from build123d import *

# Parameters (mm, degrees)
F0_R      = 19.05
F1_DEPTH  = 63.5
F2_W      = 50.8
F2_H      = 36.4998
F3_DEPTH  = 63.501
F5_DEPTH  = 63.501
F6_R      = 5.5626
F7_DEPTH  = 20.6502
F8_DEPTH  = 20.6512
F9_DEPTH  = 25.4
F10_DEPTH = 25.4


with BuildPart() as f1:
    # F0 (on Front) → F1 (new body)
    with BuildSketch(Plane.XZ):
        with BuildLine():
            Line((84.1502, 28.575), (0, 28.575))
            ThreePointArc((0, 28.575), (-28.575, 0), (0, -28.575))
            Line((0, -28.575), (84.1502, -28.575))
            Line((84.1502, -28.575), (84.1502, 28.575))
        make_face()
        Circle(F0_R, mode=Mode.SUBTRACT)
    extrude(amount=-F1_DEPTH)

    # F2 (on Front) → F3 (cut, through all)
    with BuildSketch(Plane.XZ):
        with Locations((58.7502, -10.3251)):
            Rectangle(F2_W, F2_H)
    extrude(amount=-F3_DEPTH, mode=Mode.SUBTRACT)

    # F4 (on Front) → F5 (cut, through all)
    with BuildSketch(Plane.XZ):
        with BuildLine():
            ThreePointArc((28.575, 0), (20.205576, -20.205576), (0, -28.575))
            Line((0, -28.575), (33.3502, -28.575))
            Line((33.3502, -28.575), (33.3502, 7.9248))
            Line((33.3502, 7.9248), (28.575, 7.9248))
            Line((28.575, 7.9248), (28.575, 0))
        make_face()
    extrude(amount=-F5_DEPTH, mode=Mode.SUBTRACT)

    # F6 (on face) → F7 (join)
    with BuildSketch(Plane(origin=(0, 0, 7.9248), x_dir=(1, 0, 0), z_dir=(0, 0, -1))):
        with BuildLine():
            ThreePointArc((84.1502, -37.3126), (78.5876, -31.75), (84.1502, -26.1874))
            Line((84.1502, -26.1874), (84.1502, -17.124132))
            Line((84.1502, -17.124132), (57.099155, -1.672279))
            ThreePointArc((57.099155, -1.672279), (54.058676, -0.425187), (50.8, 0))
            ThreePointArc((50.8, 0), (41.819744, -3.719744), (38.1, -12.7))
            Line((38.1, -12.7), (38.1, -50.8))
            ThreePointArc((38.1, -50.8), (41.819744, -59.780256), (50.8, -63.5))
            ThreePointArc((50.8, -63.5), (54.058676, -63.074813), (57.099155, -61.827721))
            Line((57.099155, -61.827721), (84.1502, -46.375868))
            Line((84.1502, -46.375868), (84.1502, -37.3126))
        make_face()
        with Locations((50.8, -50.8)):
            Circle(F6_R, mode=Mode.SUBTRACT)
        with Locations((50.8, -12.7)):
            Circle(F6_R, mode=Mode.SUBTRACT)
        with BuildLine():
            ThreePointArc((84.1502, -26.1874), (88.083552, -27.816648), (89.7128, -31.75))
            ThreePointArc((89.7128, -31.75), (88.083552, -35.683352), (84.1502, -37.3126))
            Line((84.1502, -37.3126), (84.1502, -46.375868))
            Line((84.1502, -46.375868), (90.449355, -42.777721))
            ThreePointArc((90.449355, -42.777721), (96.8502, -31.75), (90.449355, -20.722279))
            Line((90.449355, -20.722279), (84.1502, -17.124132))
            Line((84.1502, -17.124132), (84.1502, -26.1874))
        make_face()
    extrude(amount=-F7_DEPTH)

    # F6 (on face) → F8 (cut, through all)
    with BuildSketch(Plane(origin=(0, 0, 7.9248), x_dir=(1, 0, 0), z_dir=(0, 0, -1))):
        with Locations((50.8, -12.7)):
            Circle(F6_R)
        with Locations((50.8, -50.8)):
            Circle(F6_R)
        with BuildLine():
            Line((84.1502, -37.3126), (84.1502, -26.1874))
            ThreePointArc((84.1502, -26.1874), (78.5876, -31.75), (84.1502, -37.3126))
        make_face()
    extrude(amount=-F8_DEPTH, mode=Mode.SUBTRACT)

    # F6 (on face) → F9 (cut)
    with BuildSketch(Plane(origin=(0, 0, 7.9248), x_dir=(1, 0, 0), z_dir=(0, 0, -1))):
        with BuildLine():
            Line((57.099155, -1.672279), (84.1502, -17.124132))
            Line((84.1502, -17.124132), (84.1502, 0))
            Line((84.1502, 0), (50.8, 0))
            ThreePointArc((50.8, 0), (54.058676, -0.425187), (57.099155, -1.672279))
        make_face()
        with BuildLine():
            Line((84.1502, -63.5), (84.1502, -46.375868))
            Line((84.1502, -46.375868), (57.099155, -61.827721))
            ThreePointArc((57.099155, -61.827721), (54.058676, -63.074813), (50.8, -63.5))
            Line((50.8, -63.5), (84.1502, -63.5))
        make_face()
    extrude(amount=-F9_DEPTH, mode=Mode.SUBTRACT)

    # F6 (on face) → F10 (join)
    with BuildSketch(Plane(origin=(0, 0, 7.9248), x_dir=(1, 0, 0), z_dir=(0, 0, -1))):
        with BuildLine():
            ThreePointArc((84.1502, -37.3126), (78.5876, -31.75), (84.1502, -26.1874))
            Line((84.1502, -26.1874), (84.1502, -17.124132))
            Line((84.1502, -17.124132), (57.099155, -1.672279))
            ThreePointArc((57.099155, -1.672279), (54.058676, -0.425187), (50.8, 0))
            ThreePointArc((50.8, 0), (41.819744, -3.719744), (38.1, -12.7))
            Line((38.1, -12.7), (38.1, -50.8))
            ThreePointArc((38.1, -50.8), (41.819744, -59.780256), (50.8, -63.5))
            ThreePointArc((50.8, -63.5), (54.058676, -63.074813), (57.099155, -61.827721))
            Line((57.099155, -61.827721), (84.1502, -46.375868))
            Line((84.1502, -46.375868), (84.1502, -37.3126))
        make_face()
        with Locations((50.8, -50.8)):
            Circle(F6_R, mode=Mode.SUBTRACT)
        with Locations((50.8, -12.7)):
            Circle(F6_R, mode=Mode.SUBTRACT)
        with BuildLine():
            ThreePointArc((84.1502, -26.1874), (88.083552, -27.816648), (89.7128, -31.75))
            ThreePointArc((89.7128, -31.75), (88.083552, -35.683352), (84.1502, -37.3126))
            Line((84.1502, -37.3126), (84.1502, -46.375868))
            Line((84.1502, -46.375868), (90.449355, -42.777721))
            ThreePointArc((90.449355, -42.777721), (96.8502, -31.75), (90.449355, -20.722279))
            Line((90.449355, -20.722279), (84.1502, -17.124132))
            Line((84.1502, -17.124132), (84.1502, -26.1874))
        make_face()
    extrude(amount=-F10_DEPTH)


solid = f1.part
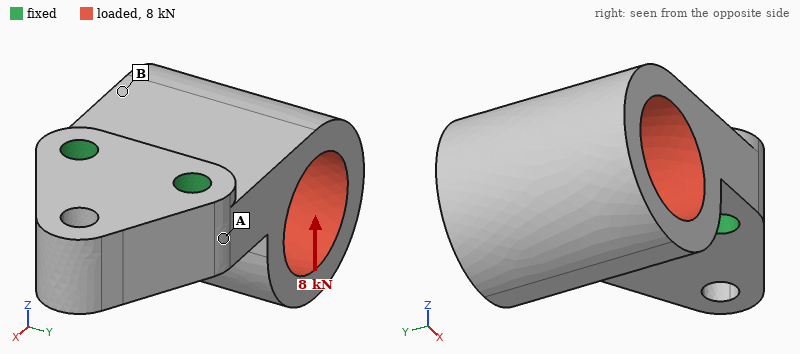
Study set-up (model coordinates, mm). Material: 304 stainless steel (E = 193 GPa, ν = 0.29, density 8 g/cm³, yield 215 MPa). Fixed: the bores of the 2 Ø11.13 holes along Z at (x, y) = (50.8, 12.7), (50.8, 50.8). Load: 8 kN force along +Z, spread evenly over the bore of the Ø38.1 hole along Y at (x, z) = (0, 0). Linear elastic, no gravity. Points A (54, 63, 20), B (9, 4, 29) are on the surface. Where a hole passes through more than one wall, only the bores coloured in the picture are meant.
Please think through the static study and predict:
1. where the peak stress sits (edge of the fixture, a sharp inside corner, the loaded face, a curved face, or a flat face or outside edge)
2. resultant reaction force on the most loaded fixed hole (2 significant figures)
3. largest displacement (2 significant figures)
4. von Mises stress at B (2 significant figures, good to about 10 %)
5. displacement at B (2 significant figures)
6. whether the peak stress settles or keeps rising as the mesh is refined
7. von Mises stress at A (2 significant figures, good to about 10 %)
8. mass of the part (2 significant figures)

edge of the fixture
4.0 kN
84 µm
42 MPa
26 µm
keeps rising
13 MPa
1.4 kg
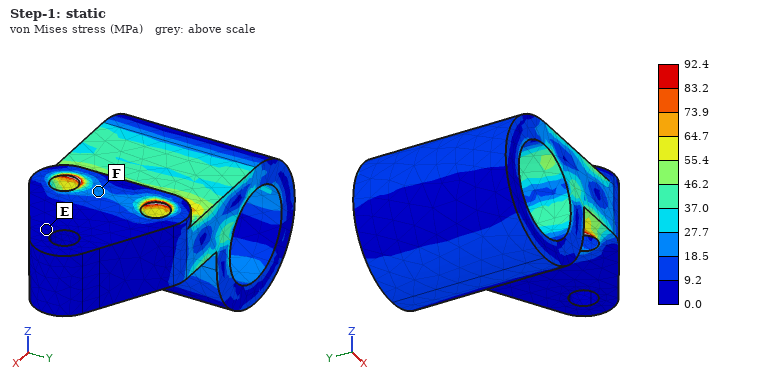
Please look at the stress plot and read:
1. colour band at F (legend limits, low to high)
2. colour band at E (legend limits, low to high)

18.5 to 27.7 MPa
0.0 to 9.2 MPa
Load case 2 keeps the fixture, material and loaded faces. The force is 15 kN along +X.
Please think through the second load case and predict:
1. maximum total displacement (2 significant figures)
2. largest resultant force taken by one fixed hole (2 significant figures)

97 µm
7.6 kN
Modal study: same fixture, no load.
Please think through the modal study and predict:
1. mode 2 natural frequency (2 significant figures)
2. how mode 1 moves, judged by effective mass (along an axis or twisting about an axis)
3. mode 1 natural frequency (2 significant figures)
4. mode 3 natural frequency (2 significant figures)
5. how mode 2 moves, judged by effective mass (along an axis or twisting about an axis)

3800 Hz
along Z
1900 Hz
6400 Hz
along Y
